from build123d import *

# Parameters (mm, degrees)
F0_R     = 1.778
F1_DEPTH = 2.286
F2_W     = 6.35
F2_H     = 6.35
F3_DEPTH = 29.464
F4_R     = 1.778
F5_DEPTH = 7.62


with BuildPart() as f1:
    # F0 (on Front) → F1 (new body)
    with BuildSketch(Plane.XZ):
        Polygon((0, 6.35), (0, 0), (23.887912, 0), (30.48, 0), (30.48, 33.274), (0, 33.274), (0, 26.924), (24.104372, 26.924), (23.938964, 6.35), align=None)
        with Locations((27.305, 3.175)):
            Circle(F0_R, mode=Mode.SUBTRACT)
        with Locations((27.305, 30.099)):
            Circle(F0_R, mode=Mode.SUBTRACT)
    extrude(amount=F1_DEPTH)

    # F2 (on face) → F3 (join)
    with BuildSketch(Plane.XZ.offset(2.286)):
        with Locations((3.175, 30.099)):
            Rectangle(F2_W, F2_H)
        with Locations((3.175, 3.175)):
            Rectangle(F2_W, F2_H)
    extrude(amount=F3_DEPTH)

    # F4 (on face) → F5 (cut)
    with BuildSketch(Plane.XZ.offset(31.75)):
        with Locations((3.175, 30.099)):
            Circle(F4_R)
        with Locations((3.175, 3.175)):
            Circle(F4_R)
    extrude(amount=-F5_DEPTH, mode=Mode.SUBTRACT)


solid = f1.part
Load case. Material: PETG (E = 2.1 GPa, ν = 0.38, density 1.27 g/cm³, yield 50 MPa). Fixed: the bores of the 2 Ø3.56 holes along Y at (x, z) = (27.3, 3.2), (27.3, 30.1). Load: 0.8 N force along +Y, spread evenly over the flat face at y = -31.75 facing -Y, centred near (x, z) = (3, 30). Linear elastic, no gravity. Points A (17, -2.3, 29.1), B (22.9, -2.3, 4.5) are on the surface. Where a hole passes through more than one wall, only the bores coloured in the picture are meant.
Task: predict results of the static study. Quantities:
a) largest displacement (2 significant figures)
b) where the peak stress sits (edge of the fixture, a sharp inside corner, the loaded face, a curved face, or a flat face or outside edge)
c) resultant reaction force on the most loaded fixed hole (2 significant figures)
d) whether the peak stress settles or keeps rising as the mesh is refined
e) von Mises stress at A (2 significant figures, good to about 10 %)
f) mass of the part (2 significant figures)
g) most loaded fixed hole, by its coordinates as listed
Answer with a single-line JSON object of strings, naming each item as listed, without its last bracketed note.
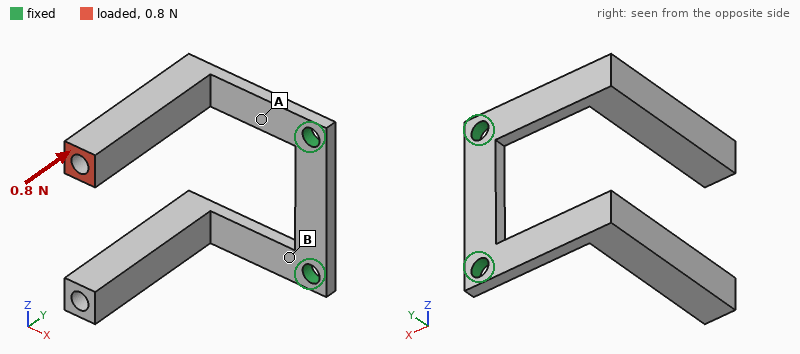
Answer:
{"largest displacement": "0.54 mm", "where the peak stress sits": "edge of the fixture", "resultant reaction force on the most loaded fixed hole": "0.86 N", "whether the peak stress settles or keeps rising as the mesh is refined": "keeps rising", "von Mises stress at A": "2.0 MPa", "mass of the part": "4.3 g", "most loaded fixed hole, by its coordinates as listed": "(27.3, 30.1)"}
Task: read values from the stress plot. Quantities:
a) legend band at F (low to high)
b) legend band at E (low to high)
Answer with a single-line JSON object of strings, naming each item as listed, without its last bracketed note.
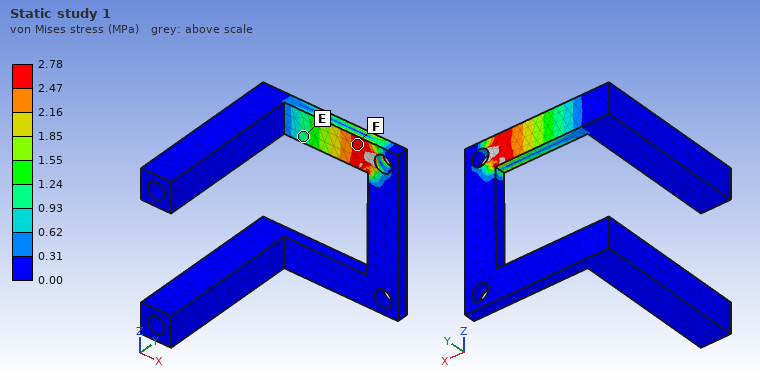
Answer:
{"legend band at F": "2.47 to 2.78 MPa", "legend band at E": "0.93 to 1.24 MPa"}
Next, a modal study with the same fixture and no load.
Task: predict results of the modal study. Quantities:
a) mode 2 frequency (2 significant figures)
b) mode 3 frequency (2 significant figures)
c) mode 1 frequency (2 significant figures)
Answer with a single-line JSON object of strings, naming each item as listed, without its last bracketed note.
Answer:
{"mode 2 frequency": "150 Hz", "mode 3 frequency": "210 Hz", "mode 1 frequency": "150 Hz"}
